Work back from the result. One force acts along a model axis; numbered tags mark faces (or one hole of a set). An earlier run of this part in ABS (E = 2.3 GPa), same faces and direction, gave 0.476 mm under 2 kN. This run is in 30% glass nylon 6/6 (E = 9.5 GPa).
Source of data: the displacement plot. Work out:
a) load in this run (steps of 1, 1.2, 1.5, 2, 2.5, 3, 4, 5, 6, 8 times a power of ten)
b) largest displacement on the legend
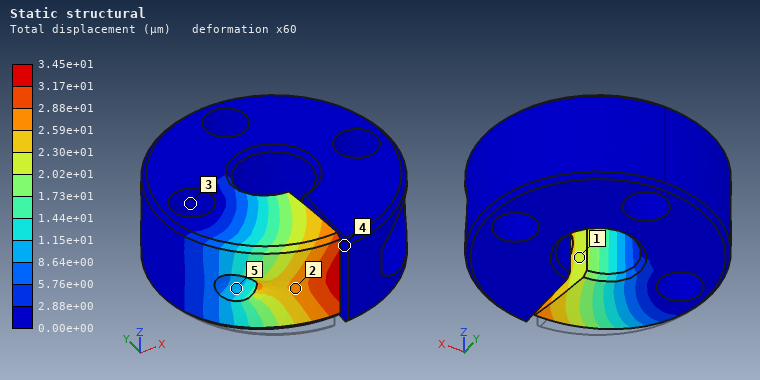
600 N
3.45e+01 µm
